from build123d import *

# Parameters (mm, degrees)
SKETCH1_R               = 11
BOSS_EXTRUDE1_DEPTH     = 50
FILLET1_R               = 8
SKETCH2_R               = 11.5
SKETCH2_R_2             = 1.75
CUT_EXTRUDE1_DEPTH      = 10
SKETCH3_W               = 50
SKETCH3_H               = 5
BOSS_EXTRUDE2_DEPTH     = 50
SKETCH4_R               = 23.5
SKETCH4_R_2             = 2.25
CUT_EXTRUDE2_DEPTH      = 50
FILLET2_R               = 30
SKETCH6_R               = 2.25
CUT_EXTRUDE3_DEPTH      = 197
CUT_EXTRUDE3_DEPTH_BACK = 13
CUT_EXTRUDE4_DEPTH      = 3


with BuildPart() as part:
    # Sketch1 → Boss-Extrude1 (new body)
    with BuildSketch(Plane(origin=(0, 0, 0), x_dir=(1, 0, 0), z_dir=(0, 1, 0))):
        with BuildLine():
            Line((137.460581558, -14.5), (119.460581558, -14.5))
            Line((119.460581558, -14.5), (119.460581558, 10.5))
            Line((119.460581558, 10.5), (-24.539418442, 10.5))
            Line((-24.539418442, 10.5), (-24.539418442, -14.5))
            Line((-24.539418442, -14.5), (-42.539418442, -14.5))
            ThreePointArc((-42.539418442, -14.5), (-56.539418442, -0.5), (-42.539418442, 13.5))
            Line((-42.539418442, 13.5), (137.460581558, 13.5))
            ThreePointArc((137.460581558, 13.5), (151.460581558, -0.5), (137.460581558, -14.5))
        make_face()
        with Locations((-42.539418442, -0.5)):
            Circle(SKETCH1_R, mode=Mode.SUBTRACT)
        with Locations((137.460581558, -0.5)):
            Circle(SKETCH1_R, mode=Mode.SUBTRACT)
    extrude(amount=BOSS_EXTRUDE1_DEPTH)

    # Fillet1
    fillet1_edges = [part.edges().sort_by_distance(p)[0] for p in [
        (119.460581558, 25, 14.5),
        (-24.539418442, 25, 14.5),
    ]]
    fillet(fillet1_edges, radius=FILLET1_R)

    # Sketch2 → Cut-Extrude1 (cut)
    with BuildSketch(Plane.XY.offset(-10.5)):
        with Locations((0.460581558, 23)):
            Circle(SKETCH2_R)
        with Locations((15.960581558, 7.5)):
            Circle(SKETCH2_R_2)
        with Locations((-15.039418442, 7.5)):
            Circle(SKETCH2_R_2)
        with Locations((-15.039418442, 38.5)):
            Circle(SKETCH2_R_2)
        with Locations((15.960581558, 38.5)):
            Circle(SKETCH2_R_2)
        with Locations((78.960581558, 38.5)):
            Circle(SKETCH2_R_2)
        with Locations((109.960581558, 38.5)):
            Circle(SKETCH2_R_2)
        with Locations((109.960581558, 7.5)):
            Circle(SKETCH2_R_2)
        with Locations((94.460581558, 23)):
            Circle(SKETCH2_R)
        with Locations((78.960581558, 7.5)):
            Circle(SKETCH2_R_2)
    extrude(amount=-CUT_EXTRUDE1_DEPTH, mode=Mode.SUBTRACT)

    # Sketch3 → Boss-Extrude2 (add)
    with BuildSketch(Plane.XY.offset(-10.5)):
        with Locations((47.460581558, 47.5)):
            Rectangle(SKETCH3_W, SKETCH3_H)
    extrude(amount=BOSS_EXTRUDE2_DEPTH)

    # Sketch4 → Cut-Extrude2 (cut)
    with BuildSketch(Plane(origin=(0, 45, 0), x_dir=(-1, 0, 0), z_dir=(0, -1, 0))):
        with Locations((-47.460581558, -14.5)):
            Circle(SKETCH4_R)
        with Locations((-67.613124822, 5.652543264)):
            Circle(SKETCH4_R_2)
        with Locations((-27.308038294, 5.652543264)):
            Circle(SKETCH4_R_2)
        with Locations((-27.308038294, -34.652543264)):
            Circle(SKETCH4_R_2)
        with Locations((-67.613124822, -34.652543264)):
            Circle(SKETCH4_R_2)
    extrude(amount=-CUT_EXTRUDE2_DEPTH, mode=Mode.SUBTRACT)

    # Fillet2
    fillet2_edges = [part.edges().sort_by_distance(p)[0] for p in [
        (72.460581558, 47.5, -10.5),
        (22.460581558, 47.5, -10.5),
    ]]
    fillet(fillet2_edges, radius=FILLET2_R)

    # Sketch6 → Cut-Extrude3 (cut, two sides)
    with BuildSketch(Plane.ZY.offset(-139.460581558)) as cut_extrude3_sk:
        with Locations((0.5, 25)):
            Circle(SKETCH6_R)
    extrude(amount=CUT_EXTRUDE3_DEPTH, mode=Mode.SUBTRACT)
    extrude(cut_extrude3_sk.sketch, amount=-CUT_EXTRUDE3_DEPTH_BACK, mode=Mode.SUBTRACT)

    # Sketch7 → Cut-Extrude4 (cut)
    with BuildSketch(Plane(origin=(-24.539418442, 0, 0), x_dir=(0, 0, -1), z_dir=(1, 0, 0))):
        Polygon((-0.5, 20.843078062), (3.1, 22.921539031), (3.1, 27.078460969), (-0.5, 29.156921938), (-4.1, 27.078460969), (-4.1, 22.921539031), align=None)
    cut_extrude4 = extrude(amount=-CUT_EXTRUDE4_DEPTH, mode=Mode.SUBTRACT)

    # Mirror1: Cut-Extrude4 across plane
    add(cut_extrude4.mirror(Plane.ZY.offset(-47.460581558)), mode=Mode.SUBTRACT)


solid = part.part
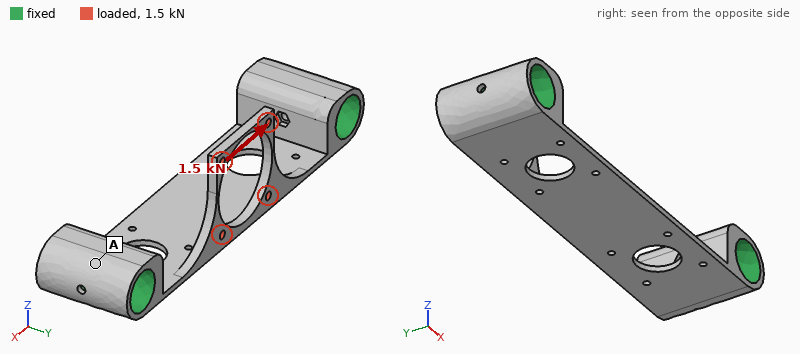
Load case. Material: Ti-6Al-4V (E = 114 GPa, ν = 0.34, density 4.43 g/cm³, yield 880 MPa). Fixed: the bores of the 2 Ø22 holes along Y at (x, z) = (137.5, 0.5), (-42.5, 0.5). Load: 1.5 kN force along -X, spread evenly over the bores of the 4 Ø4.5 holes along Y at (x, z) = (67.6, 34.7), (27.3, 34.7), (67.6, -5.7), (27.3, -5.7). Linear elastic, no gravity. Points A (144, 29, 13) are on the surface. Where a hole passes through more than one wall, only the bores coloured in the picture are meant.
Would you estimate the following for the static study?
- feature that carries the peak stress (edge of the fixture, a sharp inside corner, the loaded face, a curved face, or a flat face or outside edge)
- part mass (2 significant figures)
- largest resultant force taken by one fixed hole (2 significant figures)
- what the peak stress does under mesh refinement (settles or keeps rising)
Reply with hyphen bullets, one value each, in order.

- a sharp inside corner
- 290 g
- 840 N
- keeps rising
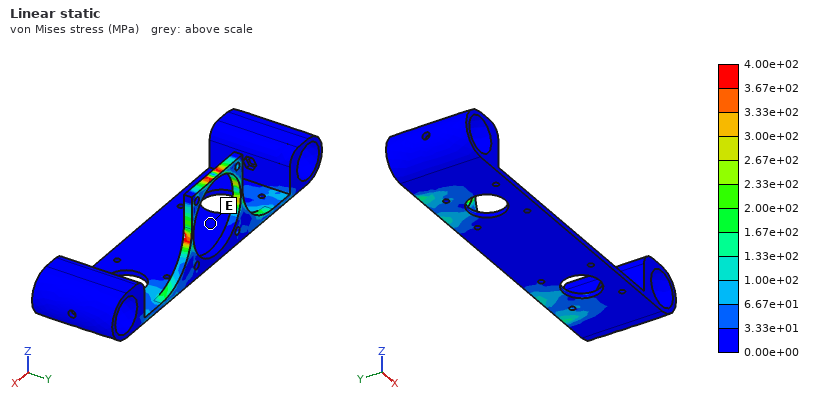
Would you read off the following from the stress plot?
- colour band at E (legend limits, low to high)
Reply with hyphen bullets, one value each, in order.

- 0.00e+00 to 3.33e+01 MPa
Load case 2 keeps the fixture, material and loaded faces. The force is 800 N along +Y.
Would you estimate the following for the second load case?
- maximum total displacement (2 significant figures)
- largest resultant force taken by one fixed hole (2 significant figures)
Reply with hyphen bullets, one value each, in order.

- 2.3 mm
- 460 N
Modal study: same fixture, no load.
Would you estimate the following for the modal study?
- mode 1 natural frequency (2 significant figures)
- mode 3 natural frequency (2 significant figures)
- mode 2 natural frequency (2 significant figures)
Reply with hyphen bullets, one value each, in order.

- 780 Hz
- 1700 Hz
- 790 Hz
